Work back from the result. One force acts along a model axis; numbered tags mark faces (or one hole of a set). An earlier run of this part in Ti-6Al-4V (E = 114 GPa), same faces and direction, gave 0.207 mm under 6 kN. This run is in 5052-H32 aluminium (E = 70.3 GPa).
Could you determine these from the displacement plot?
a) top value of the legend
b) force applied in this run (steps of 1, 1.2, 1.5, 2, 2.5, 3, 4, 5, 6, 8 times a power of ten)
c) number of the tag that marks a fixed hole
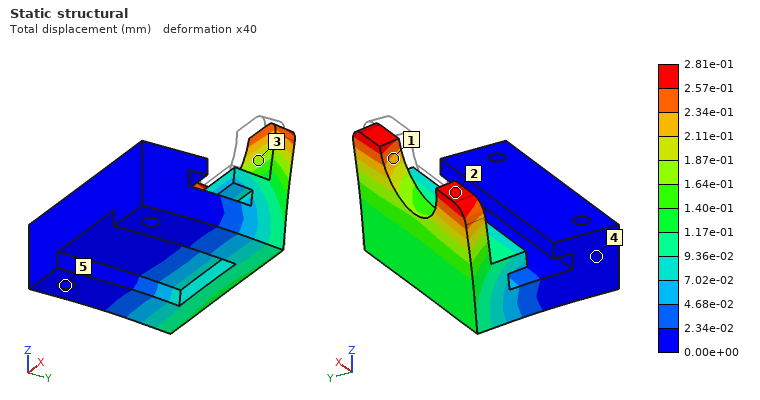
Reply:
2.81e-01 mm
5 kN
5
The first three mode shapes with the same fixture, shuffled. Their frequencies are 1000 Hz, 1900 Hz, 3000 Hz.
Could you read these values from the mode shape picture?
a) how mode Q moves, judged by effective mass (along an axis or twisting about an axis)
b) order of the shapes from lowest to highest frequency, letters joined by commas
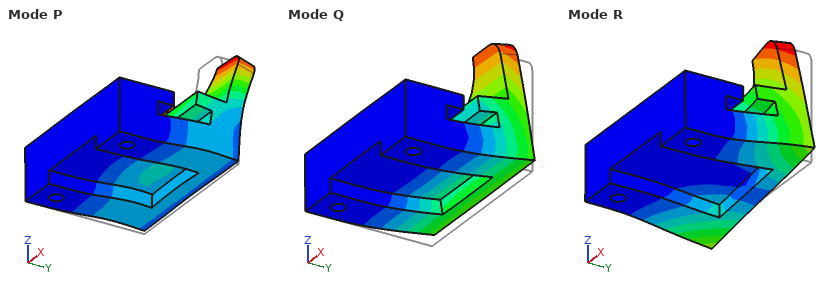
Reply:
along Z
Q, R, P
